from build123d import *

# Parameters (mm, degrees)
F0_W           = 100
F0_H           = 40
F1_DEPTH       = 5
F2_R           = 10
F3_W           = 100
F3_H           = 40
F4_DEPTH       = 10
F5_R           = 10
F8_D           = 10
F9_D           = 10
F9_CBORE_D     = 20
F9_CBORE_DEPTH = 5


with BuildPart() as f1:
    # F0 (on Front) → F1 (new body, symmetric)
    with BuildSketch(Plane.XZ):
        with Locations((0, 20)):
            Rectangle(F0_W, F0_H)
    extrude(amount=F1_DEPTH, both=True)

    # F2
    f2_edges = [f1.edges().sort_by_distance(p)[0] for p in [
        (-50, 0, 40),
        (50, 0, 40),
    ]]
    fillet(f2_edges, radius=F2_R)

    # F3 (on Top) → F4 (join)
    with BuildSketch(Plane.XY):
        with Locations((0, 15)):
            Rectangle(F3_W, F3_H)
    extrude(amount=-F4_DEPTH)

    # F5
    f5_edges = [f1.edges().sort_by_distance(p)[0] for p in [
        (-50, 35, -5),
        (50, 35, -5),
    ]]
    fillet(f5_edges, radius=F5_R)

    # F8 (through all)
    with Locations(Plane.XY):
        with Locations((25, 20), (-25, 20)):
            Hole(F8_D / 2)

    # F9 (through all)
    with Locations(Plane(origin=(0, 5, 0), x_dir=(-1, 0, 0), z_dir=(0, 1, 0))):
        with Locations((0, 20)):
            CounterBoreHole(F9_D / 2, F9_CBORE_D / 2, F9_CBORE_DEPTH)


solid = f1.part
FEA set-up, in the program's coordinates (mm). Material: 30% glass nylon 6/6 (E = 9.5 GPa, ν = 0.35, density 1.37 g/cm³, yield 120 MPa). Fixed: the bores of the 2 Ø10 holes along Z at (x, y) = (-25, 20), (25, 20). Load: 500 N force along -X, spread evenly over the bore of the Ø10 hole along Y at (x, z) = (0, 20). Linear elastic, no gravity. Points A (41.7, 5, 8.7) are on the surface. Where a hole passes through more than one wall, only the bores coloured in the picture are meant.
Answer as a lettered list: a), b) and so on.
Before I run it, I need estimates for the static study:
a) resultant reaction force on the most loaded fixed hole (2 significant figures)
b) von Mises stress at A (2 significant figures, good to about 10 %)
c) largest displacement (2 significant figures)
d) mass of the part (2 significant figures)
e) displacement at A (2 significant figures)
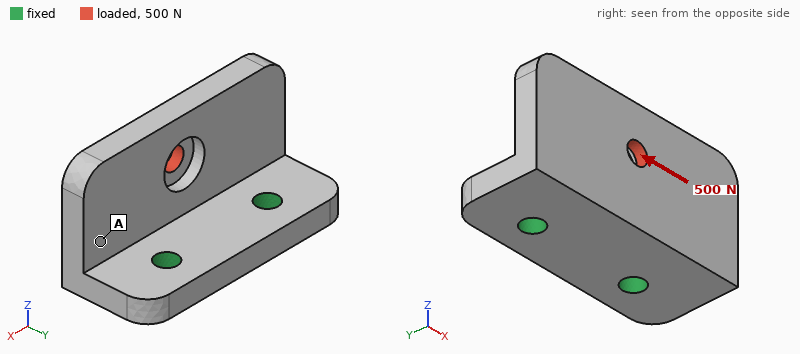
a) 370 N
b) 1.3 MPa
c) 35 µm
d) 100 g
e) 19 µm
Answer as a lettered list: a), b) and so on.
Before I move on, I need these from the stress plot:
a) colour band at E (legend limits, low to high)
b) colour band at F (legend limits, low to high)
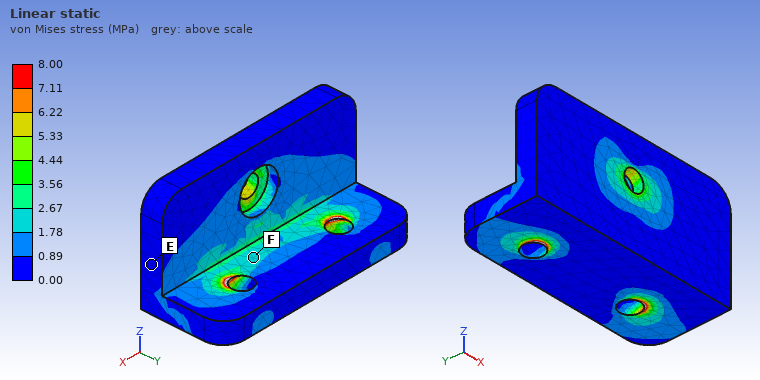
a) 0.00 to 0.89 MPa
b) 1.78 to 2.67 MPa
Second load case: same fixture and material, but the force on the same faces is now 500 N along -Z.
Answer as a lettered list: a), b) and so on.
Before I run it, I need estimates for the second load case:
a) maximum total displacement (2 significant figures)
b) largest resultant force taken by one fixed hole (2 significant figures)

a) 96 µm
b) 250 N
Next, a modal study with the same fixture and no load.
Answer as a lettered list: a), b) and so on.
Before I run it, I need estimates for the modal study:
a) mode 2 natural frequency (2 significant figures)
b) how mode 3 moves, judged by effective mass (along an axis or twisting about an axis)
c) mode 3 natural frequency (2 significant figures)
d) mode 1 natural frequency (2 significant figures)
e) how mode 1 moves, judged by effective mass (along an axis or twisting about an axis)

a) 2000 Hz
b) along X
c) 3200 Hz
d) 1300 Hz
e) along Y
